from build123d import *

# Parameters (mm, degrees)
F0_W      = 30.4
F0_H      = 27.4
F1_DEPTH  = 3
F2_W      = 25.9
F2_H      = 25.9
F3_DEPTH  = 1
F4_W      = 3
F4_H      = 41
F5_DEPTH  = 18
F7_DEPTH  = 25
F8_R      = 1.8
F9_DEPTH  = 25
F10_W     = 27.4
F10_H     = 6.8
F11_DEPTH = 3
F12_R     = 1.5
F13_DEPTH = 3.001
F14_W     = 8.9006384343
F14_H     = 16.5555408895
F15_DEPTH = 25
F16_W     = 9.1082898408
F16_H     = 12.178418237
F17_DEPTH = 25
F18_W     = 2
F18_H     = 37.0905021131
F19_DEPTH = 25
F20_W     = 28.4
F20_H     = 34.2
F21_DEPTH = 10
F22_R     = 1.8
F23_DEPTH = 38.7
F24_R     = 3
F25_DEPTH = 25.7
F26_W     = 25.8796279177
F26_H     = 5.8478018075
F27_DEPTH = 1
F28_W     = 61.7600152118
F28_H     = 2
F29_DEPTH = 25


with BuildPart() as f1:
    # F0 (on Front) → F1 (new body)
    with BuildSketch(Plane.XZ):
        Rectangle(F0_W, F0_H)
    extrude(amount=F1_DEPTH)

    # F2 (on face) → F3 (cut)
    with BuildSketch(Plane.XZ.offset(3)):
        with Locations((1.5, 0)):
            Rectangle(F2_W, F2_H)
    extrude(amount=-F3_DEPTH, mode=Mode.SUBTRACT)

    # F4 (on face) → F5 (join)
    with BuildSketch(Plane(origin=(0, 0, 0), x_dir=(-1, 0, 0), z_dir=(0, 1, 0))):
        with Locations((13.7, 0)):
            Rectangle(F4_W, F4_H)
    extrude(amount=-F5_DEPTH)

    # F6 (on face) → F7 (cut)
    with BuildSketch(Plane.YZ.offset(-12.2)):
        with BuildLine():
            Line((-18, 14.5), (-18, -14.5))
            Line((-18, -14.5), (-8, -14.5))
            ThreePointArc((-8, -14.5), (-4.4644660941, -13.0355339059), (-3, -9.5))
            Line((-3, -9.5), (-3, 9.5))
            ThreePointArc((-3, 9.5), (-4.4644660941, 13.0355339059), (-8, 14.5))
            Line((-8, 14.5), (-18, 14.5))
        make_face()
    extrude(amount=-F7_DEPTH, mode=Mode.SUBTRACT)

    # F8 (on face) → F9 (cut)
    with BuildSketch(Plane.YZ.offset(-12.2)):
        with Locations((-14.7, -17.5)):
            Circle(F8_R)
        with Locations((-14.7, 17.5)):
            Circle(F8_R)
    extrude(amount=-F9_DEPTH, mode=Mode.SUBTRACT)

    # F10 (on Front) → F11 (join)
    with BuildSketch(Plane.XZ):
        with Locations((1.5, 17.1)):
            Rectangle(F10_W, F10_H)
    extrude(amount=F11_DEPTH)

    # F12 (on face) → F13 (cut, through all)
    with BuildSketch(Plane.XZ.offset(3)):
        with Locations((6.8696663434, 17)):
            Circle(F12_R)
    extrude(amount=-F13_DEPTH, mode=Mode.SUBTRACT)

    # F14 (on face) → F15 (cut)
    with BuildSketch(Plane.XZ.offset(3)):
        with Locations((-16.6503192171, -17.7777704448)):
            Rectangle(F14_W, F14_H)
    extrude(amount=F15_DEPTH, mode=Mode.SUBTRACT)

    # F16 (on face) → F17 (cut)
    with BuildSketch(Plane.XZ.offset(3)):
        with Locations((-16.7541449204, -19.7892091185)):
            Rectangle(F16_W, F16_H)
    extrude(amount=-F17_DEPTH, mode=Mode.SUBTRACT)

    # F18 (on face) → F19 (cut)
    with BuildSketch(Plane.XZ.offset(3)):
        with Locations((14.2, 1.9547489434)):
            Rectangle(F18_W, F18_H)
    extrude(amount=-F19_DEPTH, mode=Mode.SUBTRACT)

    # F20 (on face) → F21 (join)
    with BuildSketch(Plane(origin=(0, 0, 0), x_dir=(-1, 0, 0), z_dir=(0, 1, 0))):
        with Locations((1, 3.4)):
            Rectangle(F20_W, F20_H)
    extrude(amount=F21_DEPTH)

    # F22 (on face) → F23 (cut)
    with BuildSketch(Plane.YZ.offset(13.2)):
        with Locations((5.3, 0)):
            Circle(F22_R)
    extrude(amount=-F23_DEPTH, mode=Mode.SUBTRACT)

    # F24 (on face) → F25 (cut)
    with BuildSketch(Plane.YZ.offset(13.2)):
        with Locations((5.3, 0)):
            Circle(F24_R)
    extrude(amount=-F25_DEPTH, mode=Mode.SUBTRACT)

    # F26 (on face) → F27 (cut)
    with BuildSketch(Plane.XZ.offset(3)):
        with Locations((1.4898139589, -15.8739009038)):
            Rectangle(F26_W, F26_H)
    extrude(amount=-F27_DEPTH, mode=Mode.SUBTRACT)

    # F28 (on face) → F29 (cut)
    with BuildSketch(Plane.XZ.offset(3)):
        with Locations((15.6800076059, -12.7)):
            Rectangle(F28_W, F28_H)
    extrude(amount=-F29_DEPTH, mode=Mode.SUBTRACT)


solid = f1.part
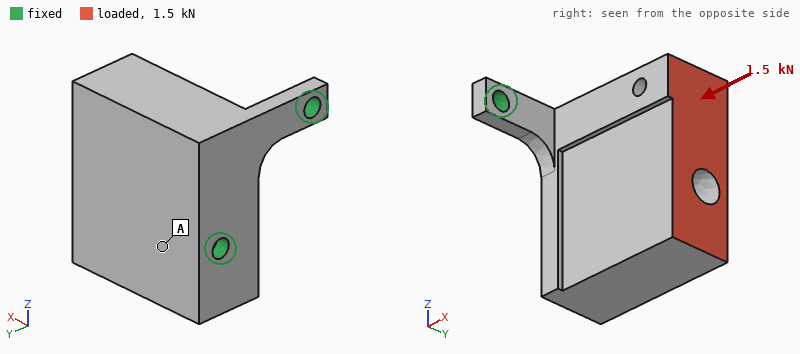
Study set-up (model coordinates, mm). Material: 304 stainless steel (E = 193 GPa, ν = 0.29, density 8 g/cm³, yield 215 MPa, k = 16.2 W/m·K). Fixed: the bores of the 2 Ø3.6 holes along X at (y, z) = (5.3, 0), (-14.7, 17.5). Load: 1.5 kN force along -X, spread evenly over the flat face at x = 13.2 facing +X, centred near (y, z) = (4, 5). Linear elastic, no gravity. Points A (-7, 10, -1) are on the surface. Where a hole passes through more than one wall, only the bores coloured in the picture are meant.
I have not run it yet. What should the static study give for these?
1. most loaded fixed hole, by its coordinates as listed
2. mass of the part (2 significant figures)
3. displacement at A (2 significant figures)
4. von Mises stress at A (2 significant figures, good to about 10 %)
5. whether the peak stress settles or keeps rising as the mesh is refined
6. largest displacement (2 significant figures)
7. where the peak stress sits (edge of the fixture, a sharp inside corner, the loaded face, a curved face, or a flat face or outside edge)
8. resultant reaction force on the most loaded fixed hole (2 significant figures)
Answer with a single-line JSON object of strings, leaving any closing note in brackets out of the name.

{"most loaded fixed hole, by its coordinates as listed": "(5.3, 0)", "mass of the part": "86 g", "displacement at A": "4.6 µm", "von Mises stress at A": "17 MPa", "whether the peak stress settles or keeps rising as the mesh is refined": "keeps rising", "largest displacement": "25 µm", "where the peak stress sits": "edge of the fixture", "resultant reaction force on the most loaded fixed hole": "1.3 kN"}
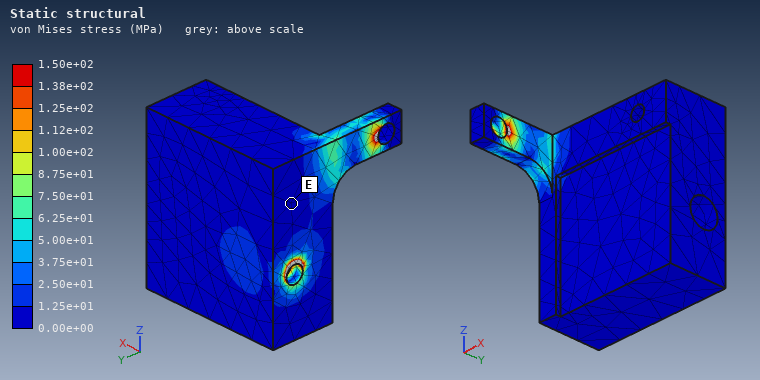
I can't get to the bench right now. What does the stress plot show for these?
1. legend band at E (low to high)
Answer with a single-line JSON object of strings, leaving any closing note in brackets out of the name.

{"legend band at E": "0.00e+00 to 1.25e+01 MPa"}
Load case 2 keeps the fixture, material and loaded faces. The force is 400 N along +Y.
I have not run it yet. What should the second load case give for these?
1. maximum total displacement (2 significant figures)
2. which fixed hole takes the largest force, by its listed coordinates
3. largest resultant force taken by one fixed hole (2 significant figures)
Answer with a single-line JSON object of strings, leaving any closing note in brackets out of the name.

{"maximum total displacement": "49 µm", "which fixed hole takes the largest force, by its listed coordinates": "(5.3, 0)", "largest resultant force taken by one fixed hole": "330 N"}
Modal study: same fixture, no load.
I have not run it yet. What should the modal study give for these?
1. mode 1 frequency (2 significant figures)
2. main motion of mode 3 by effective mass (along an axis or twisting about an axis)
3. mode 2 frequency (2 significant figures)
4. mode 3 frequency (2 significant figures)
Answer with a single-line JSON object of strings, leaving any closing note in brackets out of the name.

{"mode 1 frequency": "2400 Hz", "main motion of mode 3 by effective mass": "twisting about X", "mode 2 frequency": "3600 Hz", "mode 3 frequency": "11 kHz"}
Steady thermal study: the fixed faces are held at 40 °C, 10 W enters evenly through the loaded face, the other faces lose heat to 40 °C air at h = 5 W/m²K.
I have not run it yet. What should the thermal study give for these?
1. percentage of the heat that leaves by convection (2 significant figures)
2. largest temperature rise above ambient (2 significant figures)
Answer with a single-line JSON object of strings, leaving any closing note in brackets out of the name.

{"percentage of the heat that leaves by convection": "9.3 %", "largest temperature rise above ambient": "80 K"}
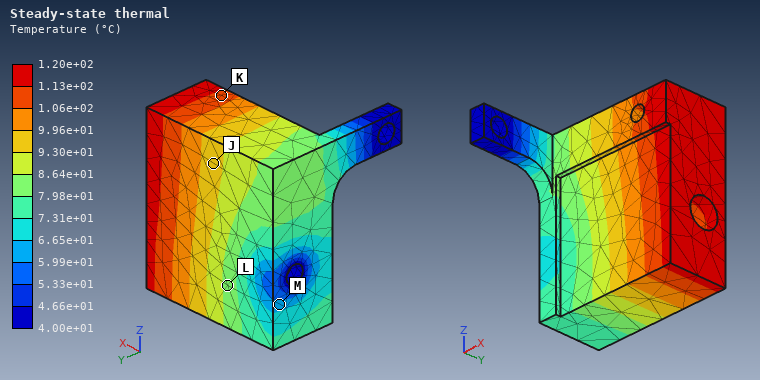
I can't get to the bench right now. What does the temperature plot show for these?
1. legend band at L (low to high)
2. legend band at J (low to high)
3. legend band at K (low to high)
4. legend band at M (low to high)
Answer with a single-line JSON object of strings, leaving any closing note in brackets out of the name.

{"legend band at L": "7.98e+01 to 8.64e+01 °C", "legend band at J": "9.30e+01 to 9.96e+01 °C", "legend band at K": "1.06e+02 to 1.13e+02 °C", "legend band at M": "5.99e+01 to 6.65e+01 °C"}
